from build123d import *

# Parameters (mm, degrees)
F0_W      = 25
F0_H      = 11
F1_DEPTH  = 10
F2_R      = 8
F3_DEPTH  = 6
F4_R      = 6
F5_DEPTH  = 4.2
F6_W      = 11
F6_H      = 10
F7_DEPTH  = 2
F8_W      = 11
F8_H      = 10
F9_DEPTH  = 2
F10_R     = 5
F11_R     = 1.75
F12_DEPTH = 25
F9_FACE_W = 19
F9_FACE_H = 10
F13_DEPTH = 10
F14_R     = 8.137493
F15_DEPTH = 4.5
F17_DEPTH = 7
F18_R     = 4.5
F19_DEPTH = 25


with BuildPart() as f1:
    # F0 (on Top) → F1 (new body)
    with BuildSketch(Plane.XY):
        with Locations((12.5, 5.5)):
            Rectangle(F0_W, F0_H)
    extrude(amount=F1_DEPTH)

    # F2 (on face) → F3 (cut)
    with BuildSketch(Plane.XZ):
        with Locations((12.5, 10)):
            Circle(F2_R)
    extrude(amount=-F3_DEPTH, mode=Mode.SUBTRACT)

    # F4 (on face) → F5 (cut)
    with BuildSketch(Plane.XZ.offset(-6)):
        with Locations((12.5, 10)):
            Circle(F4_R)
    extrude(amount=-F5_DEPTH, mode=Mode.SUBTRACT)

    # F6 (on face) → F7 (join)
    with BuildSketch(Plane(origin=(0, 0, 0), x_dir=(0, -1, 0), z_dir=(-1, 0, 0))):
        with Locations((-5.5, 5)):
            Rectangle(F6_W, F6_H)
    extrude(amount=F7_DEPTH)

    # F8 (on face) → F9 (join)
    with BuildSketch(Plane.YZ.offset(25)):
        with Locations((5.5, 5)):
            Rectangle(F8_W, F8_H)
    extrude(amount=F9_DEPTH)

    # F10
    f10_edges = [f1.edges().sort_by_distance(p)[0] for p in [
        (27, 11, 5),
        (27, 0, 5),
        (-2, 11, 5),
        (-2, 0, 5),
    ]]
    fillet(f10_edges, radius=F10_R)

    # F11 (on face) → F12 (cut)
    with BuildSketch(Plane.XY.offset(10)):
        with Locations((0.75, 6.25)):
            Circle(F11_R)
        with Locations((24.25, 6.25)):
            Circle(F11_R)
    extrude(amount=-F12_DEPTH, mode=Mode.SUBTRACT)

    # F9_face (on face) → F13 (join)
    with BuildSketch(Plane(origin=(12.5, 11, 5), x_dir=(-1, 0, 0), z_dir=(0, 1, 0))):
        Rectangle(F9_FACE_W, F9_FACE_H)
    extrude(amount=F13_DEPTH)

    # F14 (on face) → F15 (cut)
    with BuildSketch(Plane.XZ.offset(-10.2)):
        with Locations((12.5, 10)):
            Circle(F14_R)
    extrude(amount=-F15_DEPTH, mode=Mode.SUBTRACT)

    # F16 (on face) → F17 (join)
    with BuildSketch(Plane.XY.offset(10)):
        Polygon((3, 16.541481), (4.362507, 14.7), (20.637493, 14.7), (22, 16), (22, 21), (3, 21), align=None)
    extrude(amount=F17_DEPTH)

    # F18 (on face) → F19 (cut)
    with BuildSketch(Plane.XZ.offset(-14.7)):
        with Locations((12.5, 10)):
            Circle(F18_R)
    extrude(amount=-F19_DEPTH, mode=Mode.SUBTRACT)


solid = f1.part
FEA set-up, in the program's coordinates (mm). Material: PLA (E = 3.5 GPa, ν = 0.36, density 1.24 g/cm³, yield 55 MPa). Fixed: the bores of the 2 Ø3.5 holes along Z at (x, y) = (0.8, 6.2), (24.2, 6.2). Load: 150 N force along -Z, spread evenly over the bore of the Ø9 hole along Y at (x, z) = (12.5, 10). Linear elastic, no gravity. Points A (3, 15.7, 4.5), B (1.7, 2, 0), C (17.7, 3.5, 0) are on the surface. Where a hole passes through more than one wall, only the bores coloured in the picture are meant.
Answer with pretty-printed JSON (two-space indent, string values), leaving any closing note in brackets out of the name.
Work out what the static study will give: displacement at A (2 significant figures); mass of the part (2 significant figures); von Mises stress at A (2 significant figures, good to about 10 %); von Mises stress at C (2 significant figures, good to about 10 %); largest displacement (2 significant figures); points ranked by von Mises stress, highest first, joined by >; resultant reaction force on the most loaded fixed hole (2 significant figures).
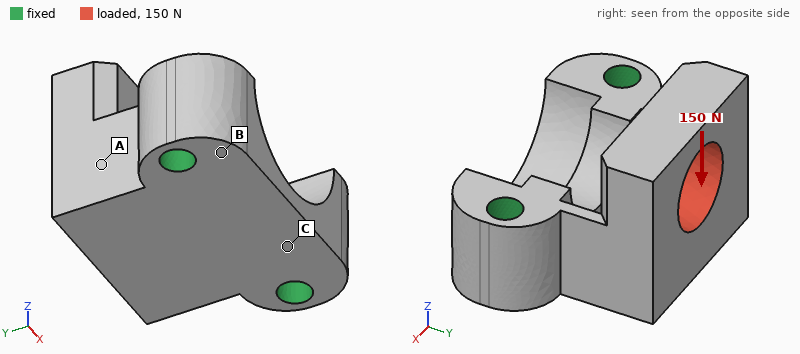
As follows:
{
  "displacement at A": "0.039 mm",
  "mass of the part": "4.7 g",
  "von Mises stress at A": "4.7 MPa",
  "von Mises stress at C": "2.3 MPa",
  "largest displacement": "0.11 mm",
  "points ranked by von Mises stress, highest first, joined by >": "A > C > B",
  "resultant reaction force on the most loaded fixed hole": "75 N"
}
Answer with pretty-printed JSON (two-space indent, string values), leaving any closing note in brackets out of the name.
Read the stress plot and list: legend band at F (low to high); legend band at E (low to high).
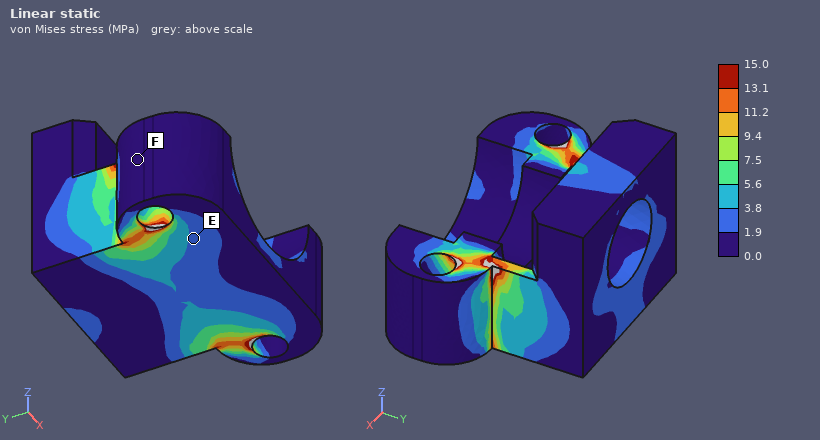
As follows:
{
  "legend band at F": "0.0 to 1.9 MPa",
  "legend band at E": "1.9 to 3.8 MPa"
}
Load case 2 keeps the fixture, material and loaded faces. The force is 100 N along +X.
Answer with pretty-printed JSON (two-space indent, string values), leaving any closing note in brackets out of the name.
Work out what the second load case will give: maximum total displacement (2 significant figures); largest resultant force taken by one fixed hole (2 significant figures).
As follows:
{
  "maximum total displacement": "75 µm",
  "largest resultant force taken by one fixed hole": "74 N"
}
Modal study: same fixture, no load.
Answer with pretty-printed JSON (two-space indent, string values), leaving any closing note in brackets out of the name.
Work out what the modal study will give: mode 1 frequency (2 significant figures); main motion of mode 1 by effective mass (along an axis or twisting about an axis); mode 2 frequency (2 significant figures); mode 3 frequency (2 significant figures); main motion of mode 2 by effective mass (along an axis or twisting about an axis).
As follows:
{
  "mode 1 frequency": "4400 Hz",
  "main motion of mode 1 by effective mass": "along Z",
  "mode 2 frequency": "5200 Hz",
  "mode 3 frequency": "8800 Hz",
  "main motion of mode 2 by effective mass": "along X"
}
